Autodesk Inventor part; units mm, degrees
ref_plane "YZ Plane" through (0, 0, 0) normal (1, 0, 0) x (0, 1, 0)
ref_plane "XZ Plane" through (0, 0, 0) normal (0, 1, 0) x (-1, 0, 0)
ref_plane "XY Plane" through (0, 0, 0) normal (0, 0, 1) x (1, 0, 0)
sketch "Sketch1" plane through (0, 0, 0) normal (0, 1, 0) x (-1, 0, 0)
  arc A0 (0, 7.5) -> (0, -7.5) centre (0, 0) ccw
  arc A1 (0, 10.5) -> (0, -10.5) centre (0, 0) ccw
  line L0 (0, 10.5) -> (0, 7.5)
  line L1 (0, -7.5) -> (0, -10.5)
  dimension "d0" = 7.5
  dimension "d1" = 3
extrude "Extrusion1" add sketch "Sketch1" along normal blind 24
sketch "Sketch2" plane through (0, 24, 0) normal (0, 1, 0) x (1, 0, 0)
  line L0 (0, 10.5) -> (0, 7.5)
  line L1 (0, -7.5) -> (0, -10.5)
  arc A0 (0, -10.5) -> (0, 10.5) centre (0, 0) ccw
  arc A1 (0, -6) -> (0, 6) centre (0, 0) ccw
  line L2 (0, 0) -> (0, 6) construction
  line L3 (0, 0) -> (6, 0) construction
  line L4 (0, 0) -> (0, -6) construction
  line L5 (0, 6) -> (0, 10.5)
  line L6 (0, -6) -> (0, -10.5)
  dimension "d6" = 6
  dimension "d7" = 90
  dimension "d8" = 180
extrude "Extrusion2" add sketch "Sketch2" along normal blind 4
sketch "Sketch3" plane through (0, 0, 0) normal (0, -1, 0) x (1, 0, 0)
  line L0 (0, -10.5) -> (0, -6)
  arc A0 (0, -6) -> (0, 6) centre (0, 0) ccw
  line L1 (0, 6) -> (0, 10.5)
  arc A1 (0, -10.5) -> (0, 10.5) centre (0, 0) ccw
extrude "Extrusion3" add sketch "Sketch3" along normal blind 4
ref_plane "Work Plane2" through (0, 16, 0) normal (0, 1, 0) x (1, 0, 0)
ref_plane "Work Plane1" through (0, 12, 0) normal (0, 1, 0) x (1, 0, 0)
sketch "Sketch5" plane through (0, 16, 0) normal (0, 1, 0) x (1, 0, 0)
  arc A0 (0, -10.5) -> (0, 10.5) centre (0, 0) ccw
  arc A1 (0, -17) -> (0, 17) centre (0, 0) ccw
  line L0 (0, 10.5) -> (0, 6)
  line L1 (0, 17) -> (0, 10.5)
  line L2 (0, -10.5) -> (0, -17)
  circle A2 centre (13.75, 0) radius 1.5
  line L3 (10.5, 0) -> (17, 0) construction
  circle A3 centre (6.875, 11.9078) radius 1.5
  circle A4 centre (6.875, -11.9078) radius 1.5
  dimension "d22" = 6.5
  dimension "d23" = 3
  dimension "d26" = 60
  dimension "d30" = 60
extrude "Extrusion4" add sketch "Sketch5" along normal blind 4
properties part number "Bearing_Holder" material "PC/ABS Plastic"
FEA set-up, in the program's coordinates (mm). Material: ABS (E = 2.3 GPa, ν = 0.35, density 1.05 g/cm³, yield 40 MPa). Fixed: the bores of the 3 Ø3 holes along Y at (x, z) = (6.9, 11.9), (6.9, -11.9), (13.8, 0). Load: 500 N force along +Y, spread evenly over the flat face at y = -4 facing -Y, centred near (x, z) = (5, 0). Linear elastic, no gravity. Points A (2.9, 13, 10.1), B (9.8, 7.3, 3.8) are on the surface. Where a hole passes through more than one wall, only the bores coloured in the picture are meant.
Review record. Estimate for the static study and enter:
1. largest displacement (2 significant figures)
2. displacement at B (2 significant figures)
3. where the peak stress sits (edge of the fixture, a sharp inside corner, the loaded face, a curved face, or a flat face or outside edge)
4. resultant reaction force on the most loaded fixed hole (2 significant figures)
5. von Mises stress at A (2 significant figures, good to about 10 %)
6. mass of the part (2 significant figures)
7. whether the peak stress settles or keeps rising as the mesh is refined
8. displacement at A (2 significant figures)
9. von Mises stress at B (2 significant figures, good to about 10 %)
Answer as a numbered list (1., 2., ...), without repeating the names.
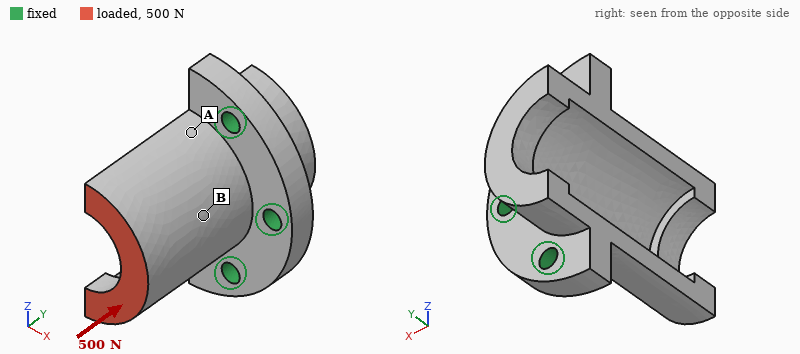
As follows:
1. 0.23 mm
2. 0.077 mm
3. edge of the fixture
4. 200 N
5. 11 MPa
6. 4.2 g
7. keeps rising
8. 0.087 mm
9. 4.8 MPa
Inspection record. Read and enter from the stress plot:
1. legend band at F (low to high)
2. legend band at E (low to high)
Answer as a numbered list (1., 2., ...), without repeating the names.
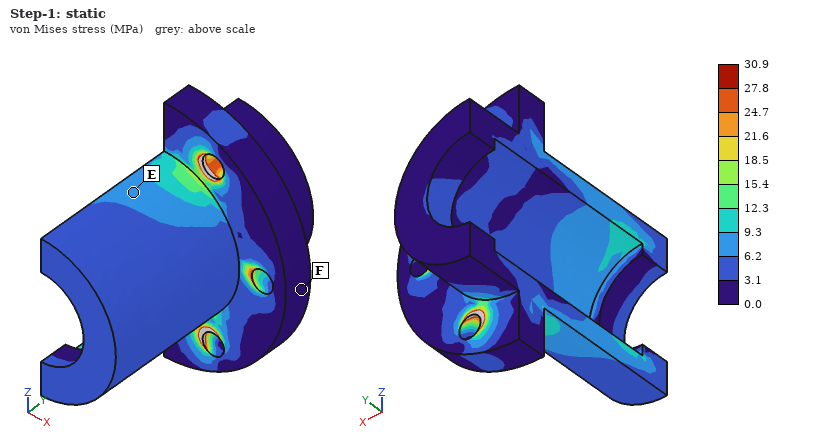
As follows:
1. 0.0 to 3.1 MPa
2. 6.2 to 9.3 MPa
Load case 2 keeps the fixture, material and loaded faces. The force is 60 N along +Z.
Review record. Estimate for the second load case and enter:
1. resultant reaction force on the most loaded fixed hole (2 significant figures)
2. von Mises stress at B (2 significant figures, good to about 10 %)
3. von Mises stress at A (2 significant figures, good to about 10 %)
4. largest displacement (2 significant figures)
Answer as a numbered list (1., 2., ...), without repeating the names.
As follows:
1. 66 N
2. 2.4 MPa
3. 6.0 MPa
4. 0.27 mm
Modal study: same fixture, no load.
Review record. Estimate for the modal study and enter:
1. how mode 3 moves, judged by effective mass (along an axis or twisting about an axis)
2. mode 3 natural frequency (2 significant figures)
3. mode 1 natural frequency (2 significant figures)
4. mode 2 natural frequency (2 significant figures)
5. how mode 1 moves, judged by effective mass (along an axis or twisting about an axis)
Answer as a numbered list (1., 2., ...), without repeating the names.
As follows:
1. along Z
2. 5100 Hz
3. 2700 Hz
4. 2900 Hz
5. along X
